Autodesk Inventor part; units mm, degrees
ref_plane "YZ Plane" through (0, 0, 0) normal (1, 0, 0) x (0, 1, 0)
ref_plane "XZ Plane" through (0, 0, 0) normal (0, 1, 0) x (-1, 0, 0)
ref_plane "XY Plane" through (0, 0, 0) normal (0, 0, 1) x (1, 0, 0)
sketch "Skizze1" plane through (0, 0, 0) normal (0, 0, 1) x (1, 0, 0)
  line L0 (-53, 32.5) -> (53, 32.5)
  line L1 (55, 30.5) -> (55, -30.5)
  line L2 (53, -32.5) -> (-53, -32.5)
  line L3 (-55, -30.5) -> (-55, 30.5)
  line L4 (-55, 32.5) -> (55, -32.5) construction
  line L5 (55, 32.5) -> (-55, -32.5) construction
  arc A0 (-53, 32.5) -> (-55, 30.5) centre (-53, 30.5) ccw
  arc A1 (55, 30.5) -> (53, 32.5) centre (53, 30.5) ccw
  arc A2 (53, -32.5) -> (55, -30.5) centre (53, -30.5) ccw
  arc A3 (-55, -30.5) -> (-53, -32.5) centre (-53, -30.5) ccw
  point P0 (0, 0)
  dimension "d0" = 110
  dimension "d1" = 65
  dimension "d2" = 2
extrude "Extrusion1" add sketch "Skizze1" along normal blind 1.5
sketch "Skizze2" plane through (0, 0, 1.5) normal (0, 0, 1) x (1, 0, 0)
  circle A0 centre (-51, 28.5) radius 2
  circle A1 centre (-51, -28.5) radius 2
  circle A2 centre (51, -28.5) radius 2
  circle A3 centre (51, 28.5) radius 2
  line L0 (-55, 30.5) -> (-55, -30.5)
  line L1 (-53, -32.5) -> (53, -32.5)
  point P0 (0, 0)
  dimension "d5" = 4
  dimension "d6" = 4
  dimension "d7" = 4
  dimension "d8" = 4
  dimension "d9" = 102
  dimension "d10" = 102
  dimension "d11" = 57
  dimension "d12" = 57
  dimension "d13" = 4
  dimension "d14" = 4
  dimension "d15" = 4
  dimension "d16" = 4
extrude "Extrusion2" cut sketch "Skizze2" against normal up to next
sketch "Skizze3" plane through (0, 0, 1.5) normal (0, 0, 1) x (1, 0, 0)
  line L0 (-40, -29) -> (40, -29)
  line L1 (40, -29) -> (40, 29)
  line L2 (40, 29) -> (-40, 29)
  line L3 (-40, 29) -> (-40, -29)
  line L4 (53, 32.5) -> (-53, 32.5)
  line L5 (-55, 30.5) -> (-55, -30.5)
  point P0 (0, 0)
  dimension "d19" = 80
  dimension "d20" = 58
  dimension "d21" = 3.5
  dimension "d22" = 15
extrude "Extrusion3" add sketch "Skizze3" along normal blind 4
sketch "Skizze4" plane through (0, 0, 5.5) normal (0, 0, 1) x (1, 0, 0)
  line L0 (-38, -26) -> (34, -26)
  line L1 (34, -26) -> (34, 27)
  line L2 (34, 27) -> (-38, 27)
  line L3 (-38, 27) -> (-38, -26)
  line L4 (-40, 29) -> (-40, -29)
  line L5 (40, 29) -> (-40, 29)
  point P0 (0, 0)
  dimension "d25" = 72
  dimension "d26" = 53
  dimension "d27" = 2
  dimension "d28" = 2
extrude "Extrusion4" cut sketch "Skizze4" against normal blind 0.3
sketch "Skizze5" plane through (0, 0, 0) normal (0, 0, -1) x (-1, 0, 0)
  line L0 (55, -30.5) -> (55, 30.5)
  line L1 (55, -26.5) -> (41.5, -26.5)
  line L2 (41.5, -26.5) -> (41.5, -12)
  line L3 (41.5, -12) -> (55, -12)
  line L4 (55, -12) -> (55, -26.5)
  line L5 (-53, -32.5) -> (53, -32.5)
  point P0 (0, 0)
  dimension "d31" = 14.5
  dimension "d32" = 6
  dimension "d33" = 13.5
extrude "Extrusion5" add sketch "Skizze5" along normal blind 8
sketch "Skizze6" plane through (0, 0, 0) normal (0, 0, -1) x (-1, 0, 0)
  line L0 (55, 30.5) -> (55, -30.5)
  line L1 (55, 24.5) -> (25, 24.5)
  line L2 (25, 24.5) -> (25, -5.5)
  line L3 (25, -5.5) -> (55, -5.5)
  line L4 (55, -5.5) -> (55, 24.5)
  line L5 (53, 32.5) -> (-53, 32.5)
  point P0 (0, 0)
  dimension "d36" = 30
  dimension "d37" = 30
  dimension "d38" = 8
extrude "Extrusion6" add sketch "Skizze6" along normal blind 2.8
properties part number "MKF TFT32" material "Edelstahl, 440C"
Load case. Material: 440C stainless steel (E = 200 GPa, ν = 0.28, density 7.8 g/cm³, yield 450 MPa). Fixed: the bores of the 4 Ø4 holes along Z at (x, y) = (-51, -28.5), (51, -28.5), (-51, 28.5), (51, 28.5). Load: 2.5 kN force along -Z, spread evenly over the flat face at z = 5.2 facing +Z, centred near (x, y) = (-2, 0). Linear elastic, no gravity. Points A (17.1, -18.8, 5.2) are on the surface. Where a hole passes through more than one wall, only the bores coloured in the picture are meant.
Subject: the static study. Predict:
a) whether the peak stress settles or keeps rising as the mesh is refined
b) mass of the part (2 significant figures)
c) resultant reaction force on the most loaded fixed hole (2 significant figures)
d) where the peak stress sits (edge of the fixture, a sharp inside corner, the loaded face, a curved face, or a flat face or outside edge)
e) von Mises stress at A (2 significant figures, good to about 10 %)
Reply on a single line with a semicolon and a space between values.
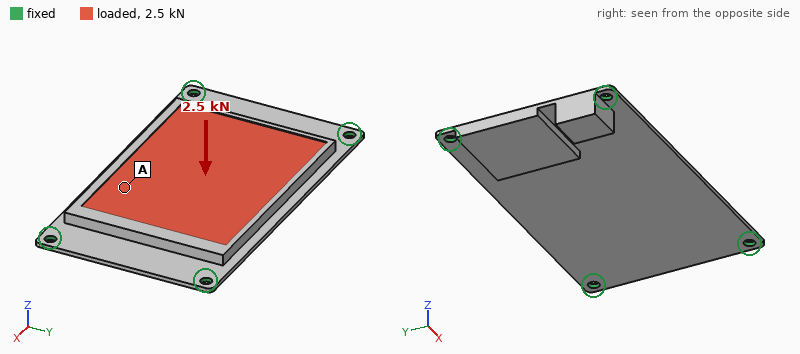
keeps rising; 250 g; 2.1 kN; edge of the fixture; 84 MPa
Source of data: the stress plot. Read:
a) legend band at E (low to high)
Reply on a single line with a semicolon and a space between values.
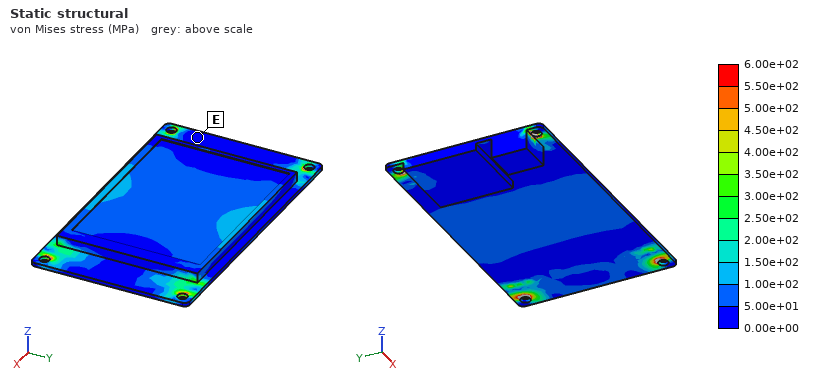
0.00e+00 to 5.00e+01 MPa
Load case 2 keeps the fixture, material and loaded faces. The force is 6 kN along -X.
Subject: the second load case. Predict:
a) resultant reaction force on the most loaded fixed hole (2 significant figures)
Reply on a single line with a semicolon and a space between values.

1.6 kN
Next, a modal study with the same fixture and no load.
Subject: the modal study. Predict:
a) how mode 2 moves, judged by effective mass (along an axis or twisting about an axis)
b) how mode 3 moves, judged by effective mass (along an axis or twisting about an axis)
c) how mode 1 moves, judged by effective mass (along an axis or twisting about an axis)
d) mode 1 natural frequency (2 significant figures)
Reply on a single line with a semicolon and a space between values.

twisting about X; twisting about Y; along Z; 1400 Hz
